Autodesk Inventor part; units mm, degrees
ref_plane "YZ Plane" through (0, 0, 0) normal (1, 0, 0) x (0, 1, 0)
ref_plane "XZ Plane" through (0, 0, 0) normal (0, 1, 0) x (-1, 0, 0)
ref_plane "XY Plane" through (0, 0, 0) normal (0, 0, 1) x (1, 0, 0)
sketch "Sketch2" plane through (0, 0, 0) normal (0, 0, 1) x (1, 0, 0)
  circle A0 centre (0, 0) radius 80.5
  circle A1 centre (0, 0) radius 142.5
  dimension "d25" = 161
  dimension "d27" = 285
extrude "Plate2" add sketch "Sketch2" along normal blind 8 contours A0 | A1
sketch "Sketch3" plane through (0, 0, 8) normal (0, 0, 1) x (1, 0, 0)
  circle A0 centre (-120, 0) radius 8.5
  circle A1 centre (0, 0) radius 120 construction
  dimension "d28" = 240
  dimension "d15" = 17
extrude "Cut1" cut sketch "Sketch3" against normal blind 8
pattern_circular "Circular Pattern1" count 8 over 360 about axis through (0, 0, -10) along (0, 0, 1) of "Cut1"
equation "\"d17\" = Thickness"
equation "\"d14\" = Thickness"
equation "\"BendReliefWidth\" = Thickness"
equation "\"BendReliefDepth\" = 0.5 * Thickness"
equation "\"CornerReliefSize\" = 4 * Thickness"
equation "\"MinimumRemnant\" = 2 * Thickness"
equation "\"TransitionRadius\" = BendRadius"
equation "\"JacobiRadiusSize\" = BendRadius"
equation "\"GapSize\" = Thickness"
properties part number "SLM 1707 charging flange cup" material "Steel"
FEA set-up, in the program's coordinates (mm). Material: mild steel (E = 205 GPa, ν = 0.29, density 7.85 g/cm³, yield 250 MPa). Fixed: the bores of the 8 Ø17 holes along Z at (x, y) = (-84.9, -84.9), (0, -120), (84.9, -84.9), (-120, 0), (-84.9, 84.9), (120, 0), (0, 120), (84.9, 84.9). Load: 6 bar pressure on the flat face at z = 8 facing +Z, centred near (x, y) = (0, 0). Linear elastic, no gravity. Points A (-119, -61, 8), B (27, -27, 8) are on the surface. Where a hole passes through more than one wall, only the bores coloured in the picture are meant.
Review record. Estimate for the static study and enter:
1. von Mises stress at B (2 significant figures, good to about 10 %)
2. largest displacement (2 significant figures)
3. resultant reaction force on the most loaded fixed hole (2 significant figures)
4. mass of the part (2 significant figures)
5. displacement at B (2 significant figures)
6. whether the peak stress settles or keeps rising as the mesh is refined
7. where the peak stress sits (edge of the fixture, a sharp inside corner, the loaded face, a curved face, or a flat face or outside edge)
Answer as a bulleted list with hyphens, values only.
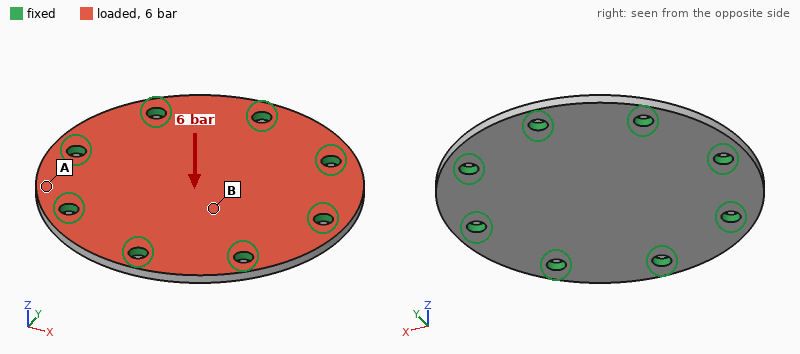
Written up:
- 51 MPa
- 0.20 mm
- 4.6 kN
- 3.9 kg
- 0.17 mm
- keeps rising
- edge of the fixture
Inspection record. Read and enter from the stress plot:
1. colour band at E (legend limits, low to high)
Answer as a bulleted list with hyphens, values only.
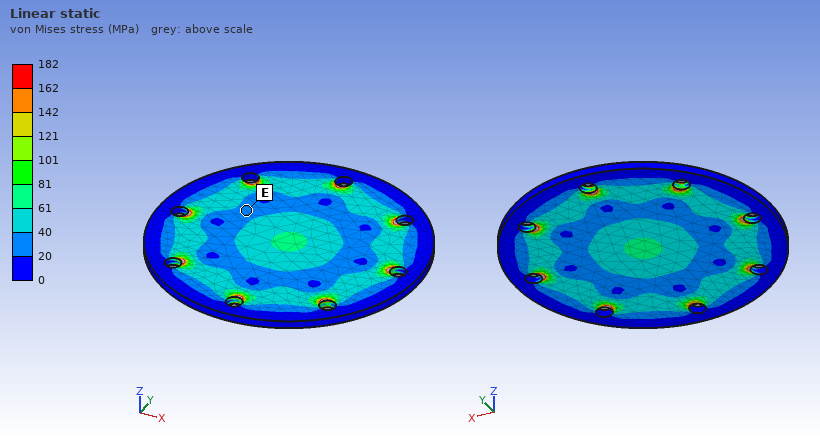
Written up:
- 20 to 40 MPa
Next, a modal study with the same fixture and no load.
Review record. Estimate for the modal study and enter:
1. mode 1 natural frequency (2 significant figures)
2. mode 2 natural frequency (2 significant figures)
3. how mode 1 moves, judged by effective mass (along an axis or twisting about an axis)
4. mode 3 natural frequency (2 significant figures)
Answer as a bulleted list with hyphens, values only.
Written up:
- 1400 Hz
- 2800 Hz
- along Z
- 2800 Hz
